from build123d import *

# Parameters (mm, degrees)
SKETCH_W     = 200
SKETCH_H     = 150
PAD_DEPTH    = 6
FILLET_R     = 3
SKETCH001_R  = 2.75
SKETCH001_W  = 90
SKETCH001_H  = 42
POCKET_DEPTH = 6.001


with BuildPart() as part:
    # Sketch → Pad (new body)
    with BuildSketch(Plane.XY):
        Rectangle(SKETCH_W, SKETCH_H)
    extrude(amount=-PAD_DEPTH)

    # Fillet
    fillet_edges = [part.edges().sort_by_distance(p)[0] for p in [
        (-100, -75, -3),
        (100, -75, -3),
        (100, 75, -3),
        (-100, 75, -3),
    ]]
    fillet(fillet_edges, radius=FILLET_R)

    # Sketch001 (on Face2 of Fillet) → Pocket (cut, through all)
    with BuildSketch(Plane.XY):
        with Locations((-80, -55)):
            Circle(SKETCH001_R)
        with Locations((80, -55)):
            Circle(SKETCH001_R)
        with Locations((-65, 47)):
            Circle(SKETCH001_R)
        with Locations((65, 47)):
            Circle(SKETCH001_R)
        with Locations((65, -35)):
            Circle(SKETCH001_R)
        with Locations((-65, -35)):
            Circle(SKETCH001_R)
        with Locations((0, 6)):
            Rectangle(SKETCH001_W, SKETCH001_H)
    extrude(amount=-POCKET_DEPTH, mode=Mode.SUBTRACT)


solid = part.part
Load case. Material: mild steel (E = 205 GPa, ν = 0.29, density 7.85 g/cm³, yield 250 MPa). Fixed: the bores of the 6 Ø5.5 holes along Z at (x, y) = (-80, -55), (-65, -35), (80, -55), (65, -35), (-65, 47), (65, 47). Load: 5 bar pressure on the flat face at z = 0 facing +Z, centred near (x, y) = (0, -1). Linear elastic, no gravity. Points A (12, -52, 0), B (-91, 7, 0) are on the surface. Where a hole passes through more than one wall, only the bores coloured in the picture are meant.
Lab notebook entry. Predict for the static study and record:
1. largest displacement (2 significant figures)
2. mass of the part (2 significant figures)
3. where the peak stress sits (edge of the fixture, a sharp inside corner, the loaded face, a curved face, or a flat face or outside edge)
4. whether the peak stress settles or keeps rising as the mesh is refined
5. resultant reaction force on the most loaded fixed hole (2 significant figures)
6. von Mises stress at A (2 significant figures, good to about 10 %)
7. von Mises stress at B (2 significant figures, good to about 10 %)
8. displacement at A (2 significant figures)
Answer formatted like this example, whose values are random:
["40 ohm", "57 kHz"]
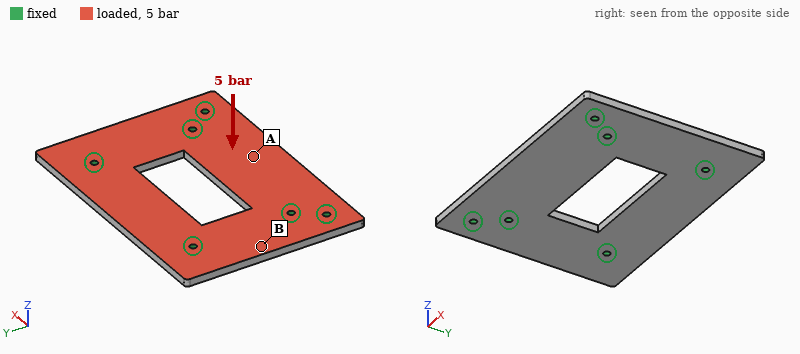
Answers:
["0.16 mm", "1.2 kg", "edge of the fixture", "keeps rising", "3.0 kN", "55 MPa", "19 MPa", "0.12 mm"]
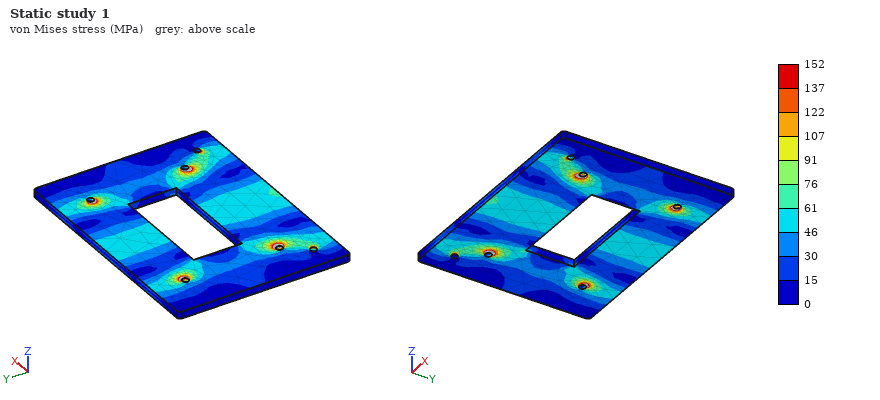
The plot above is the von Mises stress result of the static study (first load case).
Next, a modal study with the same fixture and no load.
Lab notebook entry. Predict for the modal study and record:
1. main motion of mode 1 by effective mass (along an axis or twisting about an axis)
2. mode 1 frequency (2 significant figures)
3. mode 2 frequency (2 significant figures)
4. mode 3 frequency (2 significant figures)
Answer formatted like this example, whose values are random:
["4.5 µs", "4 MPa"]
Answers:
["along Z", "1600 Hz", "1700 Hz", "2700 Hz"]
